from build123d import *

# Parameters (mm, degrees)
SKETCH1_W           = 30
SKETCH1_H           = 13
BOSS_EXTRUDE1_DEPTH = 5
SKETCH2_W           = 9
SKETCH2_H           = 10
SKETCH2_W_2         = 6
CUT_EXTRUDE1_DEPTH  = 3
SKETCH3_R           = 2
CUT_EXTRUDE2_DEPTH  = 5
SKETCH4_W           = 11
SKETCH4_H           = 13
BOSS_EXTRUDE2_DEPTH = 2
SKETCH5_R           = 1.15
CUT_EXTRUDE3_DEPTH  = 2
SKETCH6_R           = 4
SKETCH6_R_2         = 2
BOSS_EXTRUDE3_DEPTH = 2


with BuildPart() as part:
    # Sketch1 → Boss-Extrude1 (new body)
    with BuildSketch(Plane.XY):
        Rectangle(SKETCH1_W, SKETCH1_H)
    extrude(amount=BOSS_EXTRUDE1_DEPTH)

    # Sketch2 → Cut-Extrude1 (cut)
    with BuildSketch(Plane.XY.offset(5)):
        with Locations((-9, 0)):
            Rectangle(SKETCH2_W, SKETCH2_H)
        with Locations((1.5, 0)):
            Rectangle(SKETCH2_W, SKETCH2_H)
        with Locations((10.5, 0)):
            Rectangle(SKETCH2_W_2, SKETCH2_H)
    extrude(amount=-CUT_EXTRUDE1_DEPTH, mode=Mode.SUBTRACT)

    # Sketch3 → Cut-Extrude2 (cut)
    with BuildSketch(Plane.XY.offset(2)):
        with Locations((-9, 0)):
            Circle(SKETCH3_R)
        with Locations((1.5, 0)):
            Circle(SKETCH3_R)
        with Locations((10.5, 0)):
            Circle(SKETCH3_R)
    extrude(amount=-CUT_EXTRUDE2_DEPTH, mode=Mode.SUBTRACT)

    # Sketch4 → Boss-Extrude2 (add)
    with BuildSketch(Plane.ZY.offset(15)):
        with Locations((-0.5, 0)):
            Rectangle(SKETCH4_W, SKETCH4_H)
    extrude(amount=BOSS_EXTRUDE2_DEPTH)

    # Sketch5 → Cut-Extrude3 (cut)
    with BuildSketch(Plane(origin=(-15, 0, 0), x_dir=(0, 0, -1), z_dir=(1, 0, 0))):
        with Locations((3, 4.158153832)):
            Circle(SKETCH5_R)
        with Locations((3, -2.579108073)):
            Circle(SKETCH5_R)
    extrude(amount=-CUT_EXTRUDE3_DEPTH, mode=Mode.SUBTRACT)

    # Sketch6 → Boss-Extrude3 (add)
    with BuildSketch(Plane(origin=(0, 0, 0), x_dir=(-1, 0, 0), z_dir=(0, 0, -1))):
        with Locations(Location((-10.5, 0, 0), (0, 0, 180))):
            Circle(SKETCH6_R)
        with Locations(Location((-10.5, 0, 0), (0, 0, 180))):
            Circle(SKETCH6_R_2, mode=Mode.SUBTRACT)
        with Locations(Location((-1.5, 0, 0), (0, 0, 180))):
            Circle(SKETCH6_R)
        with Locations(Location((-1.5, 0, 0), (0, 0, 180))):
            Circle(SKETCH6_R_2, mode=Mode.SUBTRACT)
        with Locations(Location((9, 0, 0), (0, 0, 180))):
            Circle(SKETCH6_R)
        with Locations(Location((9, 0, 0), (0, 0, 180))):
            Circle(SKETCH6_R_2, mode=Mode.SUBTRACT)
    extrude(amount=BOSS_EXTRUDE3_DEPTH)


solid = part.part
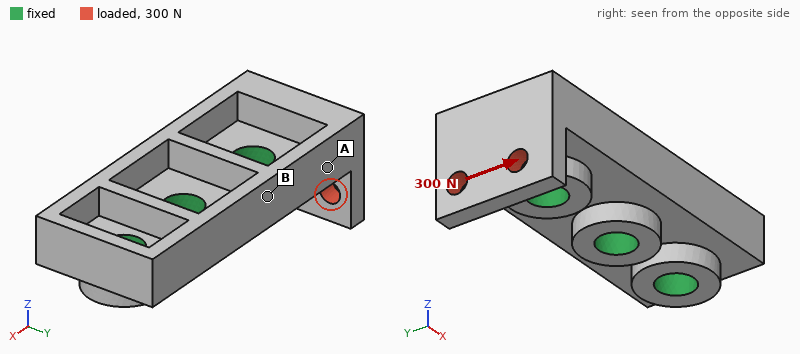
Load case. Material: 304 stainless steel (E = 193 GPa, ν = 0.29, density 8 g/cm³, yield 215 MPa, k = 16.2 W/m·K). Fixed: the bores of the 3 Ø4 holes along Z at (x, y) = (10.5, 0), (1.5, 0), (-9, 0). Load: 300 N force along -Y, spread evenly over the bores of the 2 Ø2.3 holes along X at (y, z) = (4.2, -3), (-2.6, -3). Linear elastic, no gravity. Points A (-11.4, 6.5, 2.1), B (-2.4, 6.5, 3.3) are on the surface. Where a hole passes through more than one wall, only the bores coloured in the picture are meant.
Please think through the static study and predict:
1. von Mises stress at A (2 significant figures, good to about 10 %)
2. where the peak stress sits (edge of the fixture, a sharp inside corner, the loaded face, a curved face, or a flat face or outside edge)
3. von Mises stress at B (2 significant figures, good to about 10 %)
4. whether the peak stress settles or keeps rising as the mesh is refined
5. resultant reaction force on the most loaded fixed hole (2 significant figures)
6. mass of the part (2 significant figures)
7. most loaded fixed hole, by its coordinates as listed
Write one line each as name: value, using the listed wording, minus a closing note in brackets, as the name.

von Mises stress at A: 32 MPa
where the peak stress sits: a sharp inside corner
von Mises stress at B: 9.6 MPa
whether the peak stress settles or keeps rising as the mesh is refined: keeps rising
resultant reaction force on the most loaded fixed hole: 380 N
mass of the part: 13 g
most loaded fixed hole, by its coordinates as listed: (-9, 0)
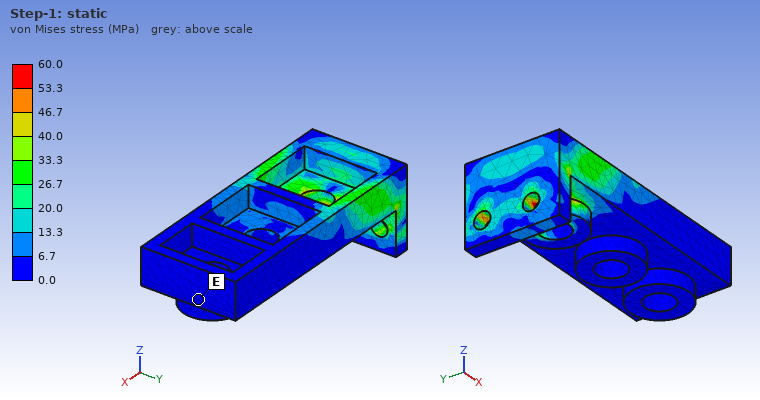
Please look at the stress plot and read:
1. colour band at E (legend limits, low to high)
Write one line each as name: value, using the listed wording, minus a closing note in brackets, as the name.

colour band at E: 0.0 to 6.7 MPa
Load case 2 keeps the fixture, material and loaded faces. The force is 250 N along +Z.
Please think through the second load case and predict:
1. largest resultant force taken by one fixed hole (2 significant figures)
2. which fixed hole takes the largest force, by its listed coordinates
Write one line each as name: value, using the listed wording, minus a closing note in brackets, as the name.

largest resultant force taken by one fixed hole: 310 N
which fixed hole takes the largest force, by its listed coordinates: (-9, 0)
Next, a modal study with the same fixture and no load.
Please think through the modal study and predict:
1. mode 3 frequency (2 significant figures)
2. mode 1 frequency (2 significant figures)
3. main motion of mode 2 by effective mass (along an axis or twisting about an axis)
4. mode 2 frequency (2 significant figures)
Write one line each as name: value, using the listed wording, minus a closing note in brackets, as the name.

mode 3 frequency: 36 kHz
mode 1 frequency: 21 kHz
main motion of mode 2 by effective mass: twisting about X
mode 2 frequency: 24 kHz
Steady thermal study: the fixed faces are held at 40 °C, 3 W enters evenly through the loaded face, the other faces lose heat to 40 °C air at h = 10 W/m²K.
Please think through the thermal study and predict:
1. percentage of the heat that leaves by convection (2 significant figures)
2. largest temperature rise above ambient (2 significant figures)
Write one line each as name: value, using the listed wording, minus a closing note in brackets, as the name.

percentage of the heat that leaves by convection: 6.2 %
largest temperature rise above ambient: 69 K
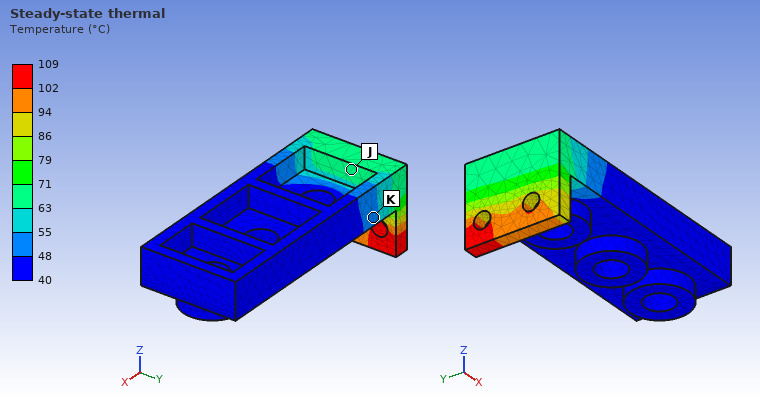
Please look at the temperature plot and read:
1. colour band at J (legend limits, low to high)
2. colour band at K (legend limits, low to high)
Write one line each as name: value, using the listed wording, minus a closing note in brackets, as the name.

colour band at J: 63 to 71 °C
colour band at K: 48 to 55 °C
